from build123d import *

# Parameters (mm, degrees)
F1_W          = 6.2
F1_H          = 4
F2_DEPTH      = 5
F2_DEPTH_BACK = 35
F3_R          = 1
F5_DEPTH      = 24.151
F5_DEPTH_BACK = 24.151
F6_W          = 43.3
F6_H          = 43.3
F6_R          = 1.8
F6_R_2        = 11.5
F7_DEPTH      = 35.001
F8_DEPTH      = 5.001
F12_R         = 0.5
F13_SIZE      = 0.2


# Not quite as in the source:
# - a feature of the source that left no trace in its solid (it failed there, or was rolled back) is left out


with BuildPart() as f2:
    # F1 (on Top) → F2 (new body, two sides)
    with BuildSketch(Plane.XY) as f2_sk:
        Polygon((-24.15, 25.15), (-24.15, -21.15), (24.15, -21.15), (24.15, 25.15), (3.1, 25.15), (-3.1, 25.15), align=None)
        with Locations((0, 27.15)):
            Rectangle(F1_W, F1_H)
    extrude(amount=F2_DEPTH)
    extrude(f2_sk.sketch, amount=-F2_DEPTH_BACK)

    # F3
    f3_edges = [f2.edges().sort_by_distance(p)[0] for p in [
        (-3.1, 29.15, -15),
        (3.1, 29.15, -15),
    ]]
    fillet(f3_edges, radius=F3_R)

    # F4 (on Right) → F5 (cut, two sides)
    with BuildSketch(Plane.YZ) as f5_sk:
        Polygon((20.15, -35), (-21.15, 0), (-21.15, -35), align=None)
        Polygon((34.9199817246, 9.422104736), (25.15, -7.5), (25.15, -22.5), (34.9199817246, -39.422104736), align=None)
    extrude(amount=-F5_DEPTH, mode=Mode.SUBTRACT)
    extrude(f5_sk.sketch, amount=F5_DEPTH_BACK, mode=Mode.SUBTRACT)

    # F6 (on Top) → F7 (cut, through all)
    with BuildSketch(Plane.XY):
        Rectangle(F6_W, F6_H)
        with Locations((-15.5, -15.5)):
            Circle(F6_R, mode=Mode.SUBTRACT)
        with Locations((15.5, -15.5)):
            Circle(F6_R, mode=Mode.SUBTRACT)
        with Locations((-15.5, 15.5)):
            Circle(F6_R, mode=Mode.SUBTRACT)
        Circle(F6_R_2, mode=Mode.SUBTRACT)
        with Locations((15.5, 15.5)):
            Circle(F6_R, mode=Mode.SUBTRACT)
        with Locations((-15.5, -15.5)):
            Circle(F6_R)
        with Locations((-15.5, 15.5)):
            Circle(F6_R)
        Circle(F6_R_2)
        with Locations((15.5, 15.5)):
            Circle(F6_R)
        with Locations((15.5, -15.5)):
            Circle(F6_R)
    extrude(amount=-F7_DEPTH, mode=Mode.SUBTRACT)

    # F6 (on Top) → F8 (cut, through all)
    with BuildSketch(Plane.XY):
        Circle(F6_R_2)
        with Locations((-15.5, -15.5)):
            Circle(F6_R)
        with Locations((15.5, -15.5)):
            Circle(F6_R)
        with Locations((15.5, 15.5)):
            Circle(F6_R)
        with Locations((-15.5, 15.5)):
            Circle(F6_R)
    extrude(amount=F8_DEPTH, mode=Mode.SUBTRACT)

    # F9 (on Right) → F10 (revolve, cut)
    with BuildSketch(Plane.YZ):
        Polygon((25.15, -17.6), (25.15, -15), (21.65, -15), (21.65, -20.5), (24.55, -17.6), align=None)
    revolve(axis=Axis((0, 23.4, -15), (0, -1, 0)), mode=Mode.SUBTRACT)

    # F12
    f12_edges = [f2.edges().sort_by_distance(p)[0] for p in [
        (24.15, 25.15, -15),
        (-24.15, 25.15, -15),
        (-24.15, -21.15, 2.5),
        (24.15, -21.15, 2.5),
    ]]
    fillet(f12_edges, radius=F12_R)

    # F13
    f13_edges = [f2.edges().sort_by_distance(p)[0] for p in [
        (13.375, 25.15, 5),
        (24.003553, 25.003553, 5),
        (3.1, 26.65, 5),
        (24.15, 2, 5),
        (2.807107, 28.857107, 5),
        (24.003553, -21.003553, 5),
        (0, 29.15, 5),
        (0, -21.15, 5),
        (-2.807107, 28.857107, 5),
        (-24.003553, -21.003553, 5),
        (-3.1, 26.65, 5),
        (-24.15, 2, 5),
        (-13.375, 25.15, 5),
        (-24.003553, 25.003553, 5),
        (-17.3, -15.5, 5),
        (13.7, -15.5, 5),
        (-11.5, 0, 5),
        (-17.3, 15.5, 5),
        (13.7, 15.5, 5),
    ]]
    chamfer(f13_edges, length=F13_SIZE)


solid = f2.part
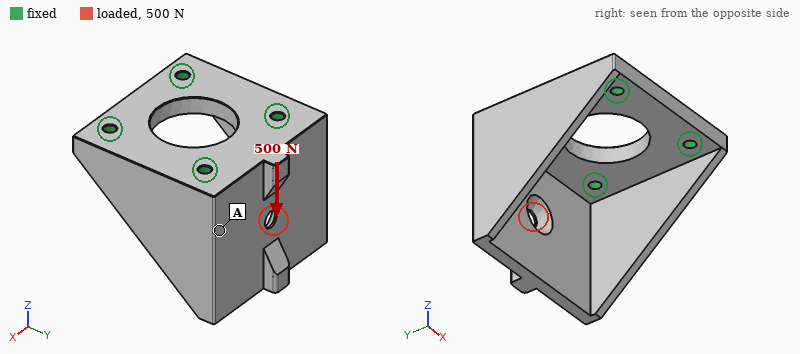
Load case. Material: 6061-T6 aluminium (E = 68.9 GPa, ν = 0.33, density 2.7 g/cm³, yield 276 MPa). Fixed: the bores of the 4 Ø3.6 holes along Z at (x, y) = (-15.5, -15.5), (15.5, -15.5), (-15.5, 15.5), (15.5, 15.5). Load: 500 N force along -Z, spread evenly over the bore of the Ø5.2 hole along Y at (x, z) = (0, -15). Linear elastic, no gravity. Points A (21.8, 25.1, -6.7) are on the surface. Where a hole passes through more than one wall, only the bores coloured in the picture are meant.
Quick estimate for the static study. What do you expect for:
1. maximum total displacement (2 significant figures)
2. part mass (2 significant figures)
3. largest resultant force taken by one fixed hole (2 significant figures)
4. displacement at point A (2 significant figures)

14 µm
51 g
300 N
3.4 µm
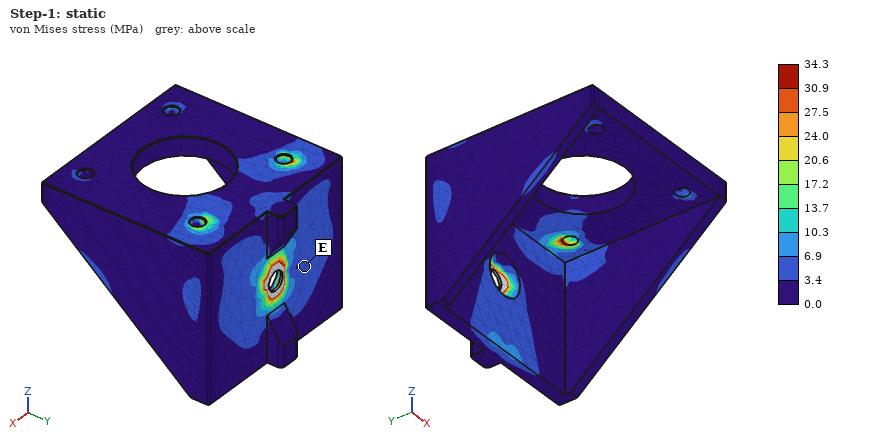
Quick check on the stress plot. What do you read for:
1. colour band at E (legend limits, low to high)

3.4 to 6.9 MPa
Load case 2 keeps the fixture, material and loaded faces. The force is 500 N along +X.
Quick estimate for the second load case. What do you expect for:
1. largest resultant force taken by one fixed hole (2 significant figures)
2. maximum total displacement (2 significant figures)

380 N
11 µm
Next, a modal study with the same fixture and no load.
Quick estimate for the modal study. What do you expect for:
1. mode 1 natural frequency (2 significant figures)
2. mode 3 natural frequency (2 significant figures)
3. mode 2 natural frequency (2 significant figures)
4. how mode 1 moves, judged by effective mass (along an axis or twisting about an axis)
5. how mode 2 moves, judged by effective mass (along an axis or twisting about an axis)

4800 Hz
9000 Hz
6900 Hz
along Y
along X
